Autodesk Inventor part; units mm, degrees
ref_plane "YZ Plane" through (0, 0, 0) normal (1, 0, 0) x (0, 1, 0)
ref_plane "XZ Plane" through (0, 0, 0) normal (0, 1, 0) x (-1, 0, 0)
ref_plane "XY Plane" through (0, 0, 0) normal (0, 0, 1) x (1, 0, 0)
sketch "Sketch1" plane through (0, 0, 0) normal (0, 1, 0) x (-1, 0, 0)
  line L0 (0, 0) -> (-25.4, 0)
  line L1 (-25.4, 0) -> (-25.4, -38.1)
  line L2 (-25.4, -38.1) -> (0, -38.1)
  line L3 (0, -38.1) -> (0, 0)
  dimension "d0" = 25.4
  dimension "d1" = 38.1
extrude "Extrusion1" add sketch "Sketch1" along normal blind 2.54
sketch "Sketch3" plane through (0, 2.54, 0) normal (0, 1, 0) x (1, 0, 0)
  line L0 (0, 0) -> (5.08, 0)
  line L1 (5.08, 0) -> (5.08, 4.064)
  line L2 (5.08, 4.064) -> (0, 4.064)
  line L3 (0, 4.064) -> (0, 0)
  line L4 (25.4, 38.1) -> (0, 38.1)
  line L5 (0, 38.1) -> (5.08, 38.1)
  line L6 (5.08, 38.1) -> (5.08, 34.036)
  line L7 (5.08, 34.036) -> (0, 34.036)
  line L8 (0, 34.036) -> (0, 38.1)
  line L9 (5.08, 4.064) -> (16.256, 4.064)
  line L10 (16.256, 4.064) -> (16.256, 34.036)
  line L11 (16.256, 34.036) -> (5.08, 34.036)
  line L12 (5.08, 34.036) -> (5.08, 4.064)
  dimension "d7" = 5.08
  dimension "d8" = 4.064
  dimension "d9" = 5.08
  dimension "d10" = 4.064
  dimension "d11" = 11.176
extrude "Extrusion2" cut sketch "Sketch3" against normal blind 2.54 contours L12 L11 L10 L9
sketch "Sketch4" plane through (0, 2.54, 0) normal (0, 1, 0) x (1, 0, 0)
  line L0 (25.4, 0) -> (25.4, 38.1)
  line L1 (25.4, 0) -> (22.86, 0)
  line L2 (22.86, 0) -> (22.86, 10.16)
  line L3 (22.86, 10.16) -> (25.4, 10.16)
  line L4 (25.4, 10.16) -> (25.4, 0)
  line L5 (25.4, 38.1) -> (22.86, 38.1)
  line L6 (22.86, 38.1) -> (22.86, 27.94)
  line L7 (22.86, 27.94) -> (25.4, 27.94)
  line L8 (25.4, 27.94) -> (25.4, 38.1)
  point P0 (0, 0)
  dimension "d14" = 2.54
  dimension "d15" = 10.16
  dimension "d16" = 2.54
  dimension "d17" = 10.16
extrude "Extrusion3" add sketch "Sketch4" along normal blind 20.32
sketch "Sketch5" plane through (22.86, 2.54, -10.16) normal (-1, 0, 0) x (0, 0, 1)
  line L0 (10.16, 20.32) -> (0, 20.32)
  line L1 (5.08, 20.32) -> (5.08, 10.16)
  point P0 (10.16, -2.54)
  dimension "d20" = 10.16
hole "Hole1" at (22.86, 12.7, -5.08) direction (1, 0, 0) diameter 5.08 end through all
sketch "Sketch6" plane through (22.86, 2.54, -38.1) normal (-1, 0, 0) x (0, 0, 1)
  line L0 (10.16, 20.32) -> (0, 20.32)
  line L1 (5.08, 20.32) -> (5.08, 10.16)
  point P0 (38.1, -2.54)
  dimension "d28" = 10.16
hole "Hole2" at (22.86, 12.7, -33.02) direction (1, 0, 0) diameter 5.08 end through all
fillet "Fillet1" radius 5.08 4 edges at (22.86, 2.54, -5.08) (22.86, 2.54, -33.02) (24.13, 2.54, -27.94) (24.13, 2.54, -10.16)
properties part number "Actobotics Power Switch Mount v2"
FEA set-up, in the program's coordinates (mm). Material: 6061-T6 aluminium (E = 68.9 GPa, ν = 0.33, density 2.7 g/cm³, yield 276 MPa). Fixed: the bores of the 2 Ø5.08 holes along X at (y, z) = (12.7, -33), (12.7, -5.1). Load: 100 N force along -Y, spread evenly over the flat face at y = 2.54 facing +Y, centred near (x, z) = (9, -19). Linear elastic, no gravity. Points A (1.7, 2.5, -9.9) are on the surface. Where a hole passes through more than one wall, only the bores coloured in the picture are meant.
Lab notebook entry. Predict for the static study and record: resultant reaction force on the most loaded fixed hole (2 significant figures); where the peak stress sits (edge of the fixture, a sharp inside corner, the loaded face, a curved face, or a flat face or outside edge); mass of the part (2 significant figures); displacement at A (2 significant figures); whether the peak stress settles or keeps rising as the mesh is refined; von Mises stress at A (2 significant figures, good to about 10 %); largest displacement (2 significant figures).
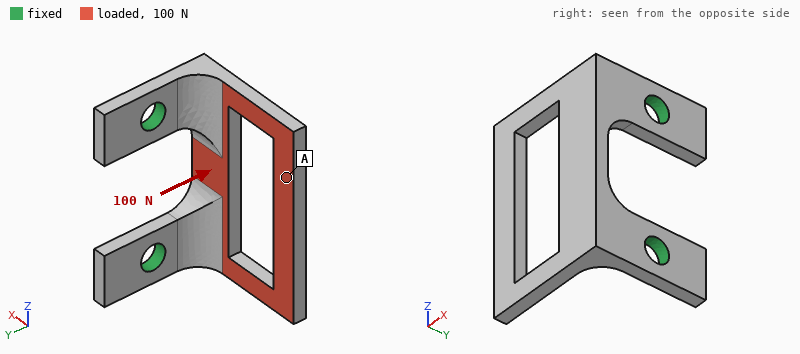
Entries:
50 N
a sharp inside corner
7.3 g
0.25 mm
keeps rising
12 MPa
0.29 mm
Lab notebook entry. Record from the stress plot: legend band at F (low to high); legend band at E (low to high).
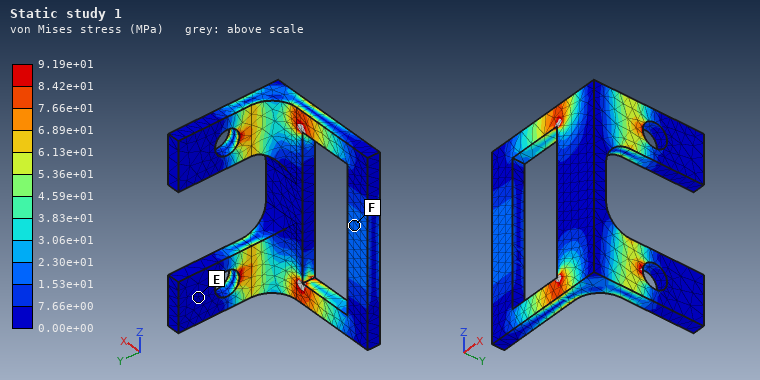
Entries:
1.53e+01 to 2.30e+01 MPa
0.00e+00 to 7.66e+00 MPa
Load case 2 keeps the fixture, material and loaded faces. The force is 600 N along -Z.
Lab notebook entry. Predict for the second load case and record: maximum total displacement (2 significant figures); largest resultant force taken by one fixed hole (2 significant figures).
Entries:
0.25 mm
400 N
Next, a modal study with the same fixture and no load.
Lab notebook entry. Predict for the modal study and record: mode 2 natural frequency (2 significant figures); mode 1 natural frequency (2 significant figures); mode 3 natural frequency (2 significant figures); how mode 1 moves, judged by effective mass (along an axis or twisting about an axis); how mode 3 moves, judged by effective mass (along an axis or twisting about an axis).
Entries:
4300 Hz
2000 Hz
6300 Hz
along Y
along Z
